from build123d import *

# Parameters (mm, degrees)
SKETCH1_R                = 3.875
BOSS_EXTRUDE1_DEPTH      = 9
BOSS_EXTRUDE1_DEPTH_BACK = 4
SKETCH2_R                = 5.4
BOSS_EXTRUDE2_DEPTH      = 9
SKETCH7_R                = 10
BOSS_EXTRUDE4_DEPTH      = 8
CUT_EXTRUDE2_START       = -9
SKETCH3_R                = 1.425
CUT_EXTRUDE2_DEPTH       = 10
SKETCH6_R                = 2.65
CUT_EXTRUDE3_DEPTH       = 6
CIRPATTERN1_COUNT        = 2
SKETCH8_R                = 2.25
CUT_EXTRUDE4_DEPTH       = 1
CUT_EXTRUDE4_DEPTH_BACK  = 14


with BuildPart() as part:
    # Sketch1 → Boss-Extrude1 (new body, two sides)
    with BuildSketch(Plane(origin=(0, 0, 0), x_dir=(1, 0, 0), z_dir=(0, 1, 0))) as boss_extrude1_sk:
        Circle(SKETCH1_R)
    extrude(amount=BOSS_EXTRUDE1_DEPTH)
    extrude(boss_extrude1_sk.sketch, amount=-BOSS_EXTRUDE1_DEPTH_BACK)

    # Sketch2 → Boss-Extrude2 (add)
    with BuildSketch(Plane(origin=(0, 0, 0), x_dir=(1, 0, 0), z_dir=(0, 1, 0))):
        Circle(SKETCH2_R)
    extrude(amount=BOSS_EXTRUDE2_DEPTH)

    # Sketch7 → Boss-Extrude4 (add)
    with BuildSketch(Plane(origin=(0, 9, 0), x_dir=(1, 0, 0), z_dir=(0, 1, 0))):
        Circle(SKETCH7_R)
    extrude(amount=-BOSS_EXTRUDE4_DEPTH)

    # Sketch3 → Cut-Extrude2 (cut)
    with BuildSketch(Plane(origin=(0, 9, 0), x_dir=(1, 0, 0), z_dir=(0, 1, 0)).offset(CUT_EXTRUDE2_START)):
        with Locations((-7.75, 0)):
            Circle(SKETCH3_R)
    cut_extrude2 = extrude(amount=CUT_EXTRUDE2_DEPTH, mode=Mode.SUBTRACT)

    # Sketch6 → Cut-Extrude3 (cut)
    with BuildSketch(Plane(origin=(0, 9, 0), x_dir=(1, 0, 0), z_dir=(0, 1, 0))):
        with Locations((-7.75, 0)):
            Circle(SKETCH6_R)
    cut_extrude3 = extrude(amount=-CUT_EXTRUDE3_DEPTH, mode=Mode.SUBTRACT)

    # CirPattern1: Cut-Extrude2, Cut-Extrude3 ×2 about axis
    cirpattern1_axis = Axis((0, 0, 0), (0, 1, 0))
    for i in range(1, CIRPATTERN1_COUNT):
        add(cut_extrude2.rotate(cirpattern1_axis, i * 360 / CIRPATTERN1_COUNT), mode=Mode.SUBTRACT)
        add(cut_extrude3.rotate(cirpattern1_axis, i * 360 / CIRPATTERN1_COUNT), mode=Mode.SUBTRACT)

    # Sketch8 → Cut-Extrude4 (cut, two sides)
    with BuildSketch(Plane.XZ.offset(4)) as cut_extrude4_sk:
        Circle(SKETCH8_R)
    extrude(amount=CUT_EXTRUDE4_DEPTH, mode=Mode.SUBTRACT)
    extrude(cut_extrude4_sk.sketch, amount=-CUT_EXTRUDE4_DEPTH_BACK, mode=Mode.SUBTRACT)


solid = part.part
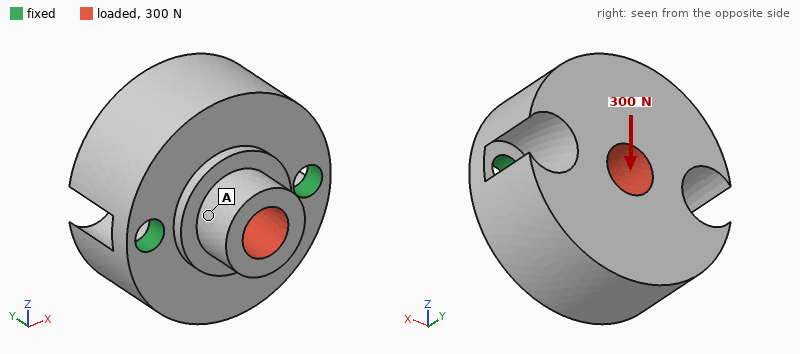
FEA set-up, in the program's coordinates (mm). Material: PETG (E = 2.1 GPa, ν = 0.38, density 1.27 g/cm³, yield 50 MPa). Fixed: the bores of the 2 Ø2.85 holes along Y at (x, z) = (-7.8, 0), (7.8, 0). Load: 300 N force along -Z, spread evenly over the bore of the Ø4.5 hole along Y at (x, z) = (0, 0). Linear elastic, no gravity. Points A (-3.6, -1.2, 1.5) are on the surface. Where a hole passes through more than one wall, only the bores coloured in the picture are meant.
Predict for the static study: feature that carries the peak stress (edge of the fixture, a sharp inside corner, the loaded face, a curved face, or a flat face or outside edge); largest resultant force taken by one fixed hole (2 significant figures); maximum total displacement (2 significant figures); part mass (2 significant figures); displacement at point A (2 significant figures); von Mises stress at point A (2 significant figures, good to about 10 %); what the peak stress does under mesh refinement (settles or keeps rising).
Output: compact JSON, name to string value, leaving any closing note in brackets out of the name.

{"feature that carries the peak stress": "edge of the fixture", "largest resultant force taken by one fixed hole": "150 N", "maximum total displacement": "90 µm", "part mass": "2.9 g", "displacement at point A": "19 µm", "von Mises stress at point A": "4.5 MPa", "what the peak stress does under mesh refinement": "keeps rising"}
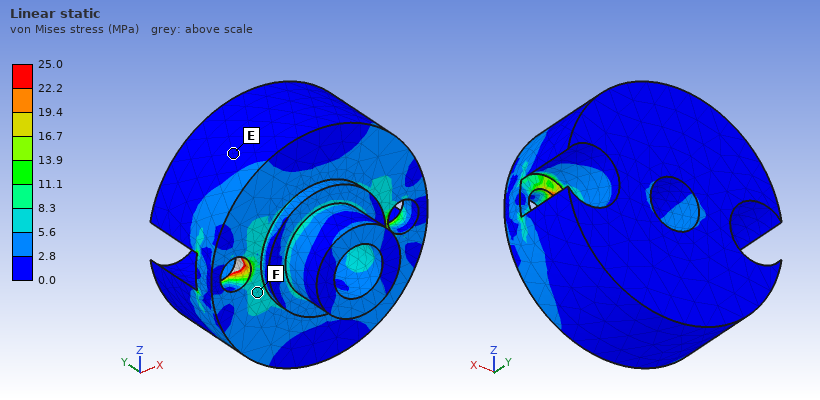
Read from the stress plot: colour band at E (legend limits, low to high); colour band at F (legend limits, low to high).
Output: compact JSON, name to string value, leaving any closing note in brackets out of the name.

{"colour band at E": "0.0 to 2.8 MPa", "colour band at F": "5.6 to 8.3 MPa"}
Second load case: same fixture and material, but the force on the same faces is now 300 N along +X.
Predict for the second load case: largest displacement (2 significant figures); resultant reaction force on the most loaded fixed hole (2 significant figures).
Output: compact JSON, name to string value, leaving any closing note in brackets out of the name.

{"largest displacement": "42 µm", "resultant reaction force on the most loaded fixed hole": "150 N"}
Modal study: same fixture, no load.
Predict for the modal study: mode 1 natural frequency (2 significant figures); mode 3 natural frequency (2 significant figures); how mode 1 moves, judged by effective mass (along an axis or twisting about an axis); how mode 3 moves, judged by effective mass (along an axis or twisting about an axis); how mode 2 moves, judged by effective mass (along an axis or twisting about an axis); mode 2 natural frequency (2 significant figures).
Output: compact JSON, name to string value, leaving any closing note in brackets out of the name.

{"mode 1 natural frequency": "2800 Hz", "mode 3 natural frequency": "10 kHz", "how mode 1 moves, judged by effective mass": "along Z", "how mode 3 moves, judged by effective mass": "along X", "how mode 2 moves, judged by effective mass": "along Y", "mode 2 natural frequency": "8200 Hz"}
